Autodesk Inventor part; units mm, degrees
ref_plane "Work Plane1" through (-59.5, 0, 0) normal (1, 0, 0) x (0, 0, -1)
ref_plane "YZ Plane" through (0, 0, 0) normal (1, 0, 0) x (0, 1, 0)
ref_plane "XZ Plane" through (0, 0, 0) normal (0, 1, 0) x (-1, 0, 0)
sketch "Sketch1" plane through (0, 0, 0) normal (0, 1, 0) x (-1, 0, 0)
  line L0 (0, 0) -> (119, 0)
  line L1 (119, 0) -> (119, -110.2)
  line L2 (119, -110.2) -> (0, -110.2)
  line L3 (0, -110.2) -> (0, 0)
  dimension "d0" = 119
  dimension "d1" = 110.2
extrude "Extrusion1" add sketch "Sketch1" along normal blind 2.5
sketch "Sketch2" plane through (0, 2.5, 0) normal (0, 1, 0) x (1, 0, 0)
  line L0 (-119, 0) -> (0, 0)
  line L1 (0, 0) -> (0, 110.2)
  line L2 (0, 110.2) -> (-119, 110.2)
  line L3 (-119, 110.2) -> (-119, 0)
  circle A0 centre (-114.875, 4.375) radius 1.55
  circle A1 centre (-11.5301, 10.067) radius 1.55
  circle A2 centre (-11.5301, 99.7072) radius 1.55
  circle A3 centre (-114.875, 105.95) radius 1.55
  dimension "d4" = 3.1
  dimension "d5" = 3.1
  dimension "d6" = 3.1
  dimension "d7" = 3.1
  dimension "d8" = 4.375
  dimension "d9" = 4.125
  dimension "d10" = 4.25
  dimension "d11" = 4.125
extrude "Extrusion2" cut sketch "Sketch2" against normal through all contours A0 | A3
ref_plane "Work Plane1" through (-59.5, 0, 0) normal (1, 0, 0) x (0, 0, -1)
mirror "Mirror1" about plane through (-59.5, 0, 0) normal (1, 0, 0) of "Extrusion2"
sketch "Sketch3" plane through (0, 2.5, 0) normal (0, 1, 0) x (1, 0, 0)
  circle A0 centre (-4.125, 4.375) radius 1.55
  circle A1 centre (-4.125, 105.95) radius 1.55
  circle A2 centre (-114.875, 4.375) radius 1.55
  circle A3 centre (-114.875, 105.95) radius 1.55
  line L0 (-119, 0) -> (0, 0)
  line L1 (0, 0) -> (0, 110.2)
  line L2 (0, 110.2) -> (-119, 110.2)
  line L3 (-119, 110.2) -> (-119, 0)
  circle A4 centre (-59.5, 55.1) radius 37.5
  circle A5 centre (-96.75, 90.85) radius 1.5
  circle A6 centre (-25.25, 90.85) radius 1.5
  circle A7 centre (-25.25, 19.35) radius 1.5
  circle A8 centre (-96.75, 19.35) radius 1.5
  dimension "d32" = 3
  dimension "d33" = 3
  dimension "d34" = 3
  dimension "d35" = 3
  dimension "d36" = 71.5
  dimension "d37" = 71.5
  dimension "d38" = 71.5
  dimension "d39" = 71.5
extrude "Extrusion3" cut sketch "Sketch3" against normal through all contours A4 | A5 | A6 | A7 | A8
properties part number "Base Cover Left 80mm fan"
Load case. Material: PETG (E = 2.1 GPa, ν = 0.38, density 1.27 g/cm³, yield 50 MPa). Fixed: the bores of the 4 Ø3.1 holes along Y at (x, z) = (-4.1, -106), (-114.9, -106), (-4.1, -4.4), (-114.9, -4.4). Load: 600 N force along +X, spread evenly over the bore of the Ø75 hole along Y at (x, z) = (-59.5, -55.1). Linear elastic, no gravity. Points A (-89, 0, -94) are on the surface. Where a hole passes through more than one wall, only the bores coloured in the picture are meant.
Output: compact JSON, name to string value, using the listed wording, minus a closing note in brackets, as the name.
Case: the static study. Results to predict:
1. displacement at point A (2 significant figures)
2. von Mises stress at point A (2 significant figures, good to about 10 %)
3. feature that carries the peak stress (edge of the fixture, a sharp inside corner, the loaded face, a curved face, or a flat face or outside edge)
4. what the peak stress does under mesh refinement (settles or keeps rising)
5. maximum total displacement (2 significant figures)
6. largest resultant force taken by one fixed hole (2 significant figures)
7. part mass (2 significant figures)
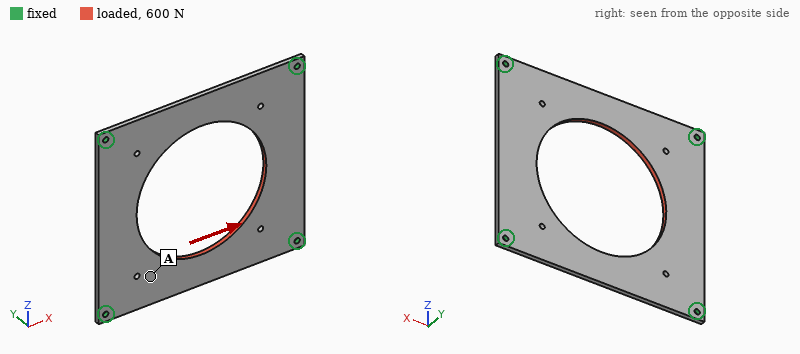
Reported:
{"displacement at point A": "0.079 mm", "von Mises stress at point A": "1.4 MPa", "feature that carries the peak stress": "edge of the fixture", "what the peak stress does under mesh refinement": "keeps rising", "maximum total displacement": "0.17 mm", "largest resultant force taken by one fixed hole": "170 N", "part mass": "27 g"}
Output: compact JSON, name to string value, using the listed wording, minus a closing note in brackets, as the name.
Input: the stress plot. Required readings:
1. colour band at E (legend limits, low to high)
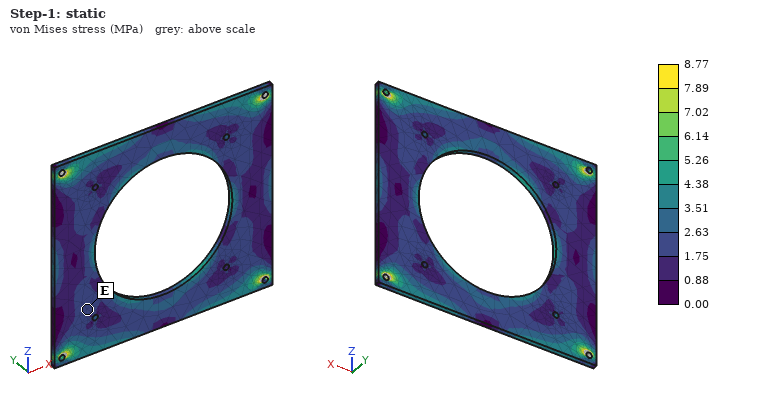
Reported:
{"colour band at E": "1.75 to 2.63 MPa"}
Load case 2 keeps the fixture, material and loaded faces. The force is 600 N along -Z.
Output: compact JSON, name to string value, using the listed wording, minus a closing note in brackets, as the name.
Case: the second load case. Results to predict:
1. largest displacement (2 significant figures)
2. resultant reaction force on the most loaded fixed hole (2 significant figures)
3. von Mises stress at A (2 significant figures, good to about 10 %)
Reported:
{"largest displacement": "0.20 mm", "resultant reaction force on the most loaded fixed hole": "170 N", "von Mises stress at A": "2.0 MPa"}
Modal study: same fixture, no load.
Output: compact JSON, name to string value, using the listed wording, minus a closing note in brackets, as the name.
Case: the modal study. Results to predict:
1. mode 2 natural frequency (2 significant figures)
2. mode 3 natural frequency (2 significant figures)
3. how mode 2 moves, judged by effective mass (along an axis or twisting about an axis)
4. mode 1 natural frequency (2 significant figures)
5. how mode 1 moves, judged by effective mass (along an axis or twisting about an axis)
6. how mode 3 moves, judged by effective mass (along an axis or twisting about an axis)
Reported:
{"mode 2 natural frequency": "290 Hz", "mode 3 natural frequency": "310 Hz", "how mode 2 moves, judged by effective mass": "twisting about X", "mode 1 natural frequency": "220 Hz", "how mode 1 moves, judged by effective mass": "along Y", "how mode 3 moves, judged by effective mass": "twisting about Z"}
